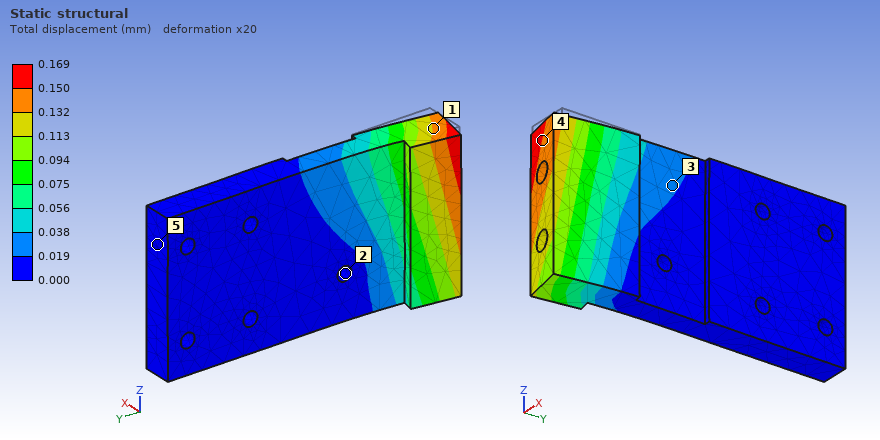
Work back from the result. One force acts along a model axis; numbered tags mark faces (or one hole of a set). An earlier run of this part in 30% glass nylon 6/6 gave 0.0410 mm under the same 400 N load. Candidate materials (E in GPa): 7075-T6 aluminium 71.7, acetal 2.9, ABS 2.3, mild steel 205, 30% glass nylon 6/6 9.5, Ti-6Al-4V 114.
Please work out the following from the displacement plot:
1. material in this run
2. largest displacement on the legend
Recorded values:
ABS
0.169 mm
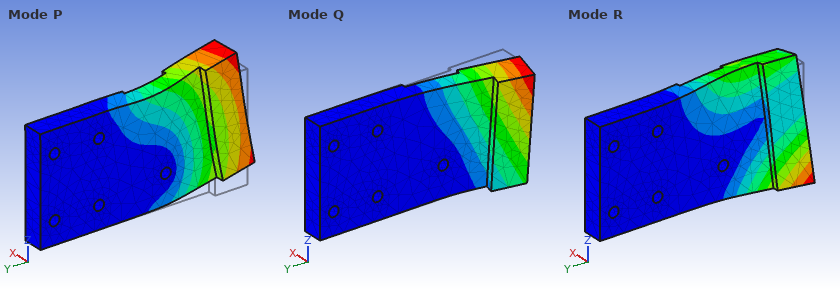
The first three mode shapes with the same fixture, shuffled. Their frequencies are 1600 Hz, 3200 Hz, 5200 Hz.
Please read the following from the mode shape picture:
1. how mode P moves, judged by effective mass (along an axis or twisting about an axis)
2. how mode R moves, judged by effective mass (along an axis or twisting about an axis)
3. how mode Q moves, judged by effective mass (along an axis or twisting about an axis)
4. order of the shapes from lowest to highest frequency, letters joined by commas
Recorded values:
along Z
twisting about Y
along X
Q, R, P
